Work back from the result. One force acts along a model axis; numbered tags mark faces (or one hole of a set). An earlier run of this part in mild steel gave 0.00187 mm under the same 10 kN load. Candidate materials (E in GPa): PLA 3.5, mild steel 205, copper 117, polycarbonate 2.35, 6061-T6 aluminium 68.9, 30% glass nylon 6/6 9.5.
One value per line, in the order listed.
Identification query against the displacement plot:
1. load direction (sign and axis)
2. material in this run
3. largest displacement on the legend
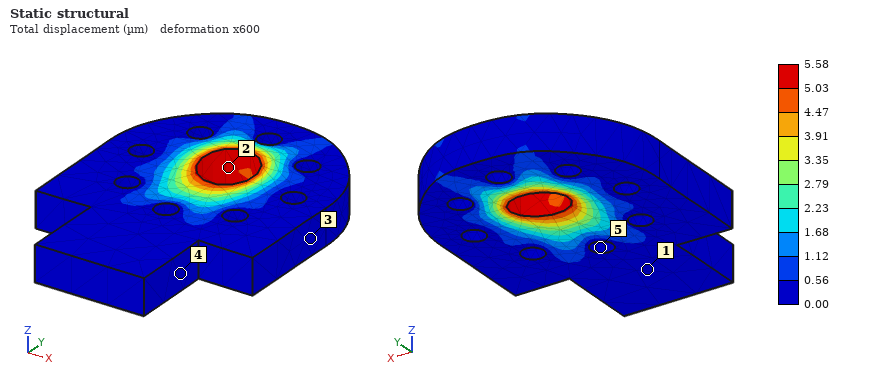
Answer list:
+Y
6061-T6 aluminium
5.58 µm
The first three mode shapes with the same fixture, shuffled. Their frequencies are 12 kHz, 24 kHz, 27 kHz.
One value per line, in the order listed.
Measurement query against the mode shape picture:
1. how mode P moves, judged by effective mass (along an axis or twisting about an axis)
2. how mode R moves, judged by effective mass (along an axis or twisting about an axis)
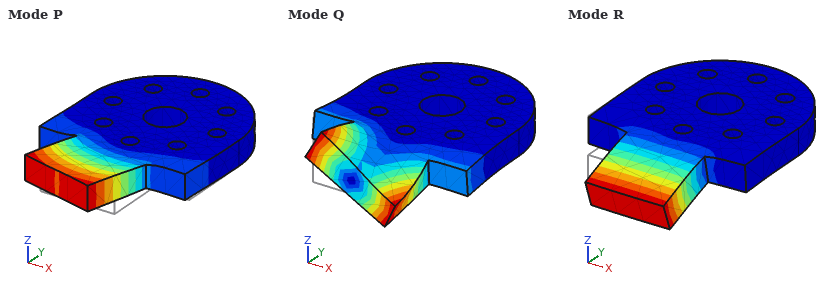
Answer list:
along X
along Z
